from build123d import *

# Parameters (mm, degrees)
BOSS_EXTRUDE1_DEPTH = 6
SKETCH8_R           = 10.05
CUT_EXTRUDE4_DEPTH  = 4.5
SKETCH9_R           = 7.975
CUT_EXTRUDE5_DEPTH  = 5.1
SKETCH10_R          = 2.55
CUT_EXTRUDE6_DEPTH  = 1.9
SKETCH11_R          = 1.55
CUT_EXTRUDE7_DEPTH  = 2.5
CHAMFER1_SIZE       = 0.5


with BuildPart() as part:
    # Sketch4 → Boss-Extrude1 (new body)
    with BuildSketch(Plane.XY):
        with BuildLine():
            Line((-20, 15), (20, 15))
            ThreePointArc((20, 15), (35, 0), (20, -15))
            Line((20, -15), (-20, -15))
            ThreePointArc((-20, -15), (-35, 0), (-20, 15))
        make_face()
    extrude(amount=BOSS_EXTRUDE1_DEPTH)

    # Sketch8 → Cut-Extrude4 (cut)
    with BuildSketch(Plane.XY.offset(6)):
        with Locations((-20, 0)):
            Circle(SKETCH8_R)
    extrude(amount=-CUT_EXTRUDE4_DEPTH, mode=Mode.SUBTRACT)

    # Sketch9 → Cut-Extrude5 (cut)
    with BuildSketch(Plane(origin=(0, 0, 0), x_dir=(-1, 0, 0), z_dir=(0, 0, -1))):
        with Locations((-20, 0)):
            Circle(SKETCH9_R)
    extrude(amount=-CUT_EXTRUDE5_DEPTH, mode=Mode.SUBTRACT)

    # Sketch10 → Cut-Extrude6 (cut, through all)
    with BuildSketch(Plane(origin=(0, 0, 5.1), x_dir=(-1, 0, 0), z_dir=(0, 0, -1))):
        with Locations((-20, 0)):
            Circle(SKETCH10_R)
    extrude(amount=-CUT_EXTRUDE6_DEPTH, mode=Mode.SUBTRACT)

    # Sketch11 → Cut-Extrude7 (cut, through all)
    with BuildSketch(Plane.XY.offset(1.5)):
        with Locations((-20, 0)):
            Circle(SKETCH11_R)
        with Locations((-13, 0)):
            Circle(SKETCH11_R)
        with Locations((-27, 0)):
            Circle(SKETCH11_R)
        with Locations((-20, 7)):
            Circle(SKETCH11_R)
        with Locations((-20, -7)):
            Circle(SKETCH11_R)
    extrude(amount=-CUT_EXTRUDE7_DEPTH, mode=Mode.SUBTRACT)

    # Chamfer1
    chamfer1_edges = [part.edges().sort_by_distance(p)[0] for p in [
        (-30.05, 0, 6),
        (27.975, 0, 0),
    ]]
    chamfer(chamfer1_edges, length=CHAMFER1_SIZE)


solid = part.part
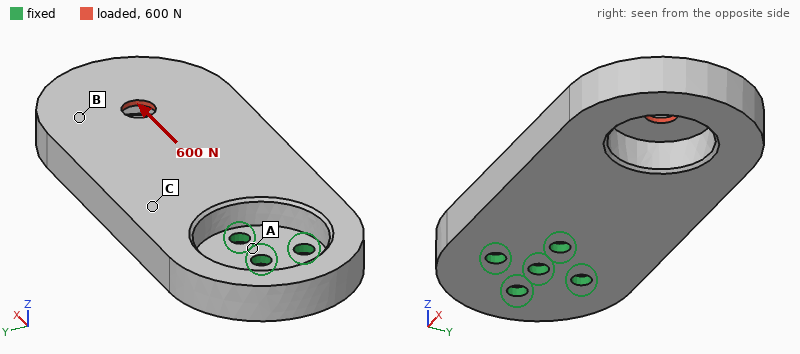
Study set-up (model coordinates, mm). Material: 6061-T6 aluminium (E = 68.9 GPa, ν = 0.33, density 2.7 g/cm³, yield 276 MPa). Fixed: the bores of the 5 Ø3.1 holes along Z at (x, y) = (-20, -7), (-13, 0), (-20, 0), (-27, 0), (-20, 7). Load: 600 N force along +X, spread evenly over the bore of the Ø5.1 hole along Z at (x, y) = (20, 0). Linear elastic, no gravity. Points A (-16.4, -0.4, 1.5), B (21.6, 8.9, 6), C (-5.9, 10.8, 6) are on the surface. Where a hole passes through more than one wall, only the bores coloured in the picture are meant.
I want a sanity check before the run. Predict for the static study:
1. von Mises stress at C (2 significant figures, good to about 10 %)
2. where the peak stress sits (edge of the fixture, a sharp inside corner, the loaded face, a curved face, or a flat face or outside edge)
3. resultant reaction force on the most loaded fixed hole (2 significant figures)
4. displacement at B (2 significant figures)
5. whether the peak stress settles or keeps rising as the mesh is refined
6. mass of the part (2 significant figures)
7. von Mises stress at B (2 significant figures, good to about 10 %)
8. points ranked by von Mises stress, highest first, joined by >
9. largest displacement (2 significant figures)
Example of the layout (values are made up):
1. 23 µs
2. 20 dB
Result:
1. 17 MPa
2. edge of the fixture
3. 260 N
4. 0.076 mm
5. keeps rising
6. 24 g
7. 9.9 MPa
8. C > B > A
9. 0.11 mm
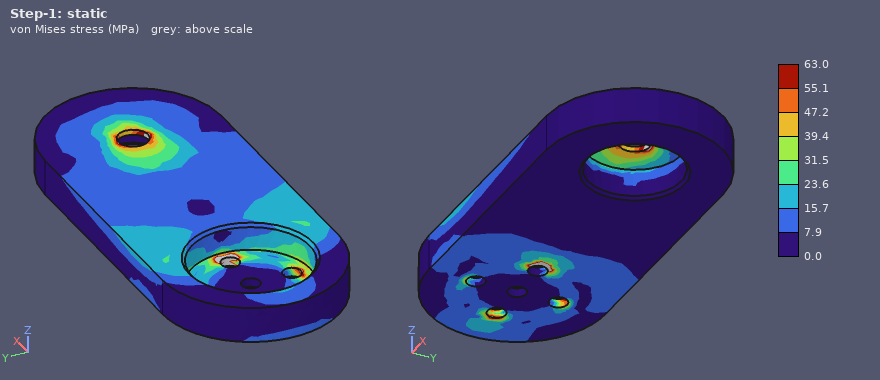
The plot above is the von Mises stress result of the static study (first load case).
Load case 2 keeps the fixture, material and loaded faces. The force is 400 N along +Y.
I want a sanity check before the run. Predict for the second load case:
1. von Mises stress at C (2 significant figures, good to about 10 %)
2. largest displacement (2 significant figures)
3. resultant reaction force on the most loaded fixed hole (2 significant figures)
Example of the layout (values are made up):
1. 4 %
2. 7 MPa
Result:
1. 11 MPa
2. 42 µm
3. 620 N
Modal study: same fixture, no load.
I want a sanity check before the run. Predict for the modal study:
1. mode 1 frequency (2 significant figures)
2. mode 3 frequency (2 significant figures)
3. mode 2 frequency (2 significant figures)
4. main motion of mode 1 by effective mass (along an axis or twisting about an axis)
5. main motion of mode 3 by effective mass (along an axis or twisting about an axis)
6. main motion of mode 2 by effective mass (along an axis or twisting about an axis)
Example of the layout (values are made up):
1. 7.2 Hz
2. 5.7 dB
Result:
1. 1600 Hz
2. 5600 Hz
3. 4800 Hz
4. along Z
5. along Y
6. twisting about X
